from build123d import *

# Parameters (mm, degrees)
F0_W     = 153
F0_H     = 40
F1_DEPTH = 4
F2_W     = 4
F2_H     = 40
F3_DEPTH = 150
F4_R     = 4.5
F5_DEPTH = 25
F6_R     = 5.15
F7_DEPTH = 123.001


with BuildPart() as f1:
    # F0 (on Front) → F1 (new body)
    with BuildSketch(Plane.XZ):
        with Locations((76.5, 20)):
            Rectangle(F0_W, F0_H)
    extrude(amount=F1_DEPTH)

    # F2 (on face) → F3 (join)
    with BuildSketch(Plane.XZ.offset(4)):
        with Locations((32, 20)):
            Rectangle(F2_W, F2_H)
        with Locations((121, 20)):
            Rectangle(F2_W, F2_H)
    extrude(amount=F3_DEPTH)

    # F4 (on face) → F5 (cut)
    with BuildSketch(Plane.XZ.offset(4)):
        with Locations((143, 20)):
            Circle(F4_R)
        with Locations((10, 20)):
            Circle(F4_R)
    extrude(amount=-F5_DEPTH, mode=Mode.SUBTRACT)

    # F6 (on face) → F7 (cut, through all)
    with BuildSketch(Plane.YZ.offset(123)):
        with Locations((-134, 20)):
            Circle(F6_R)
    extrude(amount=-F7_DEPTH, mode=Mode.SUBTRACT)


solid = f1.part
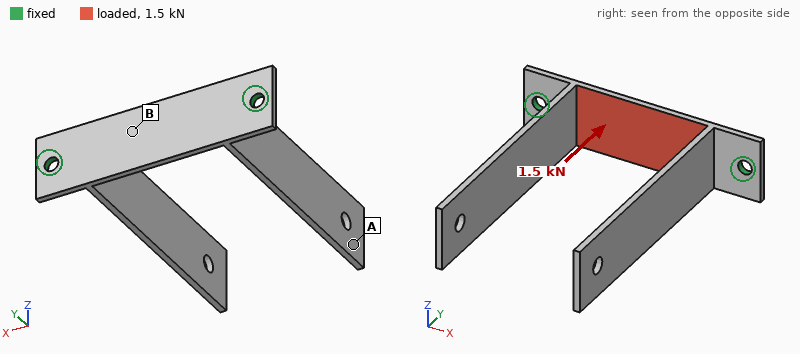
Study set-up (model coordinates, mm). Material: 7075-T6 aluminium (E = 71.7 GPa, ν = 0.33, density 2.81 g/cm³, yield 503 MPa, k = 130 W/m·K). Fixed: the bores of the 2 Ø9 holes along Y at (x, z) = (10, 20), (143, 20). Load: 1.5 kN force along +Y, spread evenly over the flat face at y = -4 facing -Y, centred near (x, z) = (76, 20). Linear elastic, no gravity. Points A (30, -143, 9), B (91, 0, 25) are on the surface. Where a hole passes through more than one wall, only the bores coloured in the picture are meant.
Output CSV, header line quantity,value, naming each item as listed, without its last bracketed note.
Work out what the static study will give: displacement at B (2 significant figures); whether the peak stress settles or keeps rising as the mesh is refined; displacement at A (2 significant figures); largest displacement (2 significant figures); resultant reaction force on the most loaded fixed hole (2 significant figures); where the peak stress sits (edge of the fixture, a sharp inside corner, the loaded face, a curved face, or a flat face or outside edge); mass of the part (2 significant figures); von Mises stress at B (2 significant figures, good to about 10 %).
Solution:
quantity,value
displacement at B,0.69 mm
whether the peak stress settles or keeps rising as the mesh is refined,keeps rising
displacement at A,2.4 mm
largest displacement,2.6 mm
resultant reaction force on the most loaded fixed hole,750 N
where the peak stress sits,edge of the fixture
mass of the part,200 g
von Mises stress at B,87 MPa
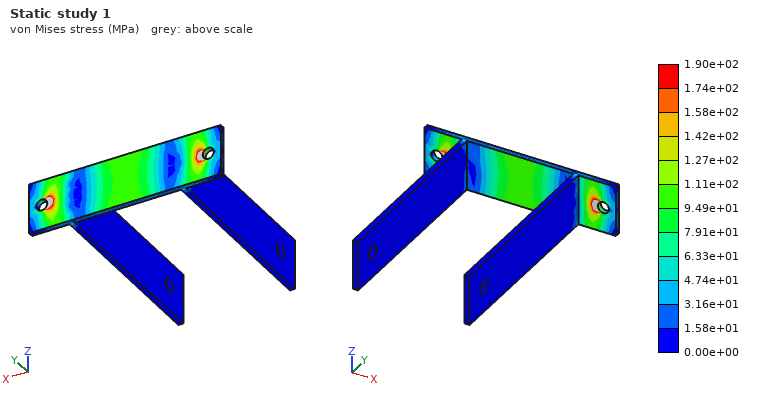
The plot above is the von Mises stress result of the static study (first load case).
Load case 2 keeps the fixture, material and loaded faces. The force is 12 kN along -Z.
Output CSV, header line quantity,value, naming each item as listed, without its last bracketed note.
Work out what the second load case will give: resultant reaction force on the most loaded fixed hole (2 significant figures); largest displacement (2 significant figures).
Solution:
quantity,value
resultant reaction force on the most loaded fixed hole,6.0 kN
largest displacement,1.4 mm
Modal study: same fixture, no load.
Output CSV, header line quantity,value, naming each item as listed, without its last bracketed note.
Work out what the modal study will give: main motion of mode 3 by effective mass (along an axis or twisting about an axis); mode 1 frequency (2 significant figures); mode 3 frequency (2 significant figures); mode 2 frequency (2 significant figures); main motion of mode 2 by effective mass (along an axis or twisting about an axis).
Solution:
quantity,value
main motion of mode 3 by effective mass,along Z
mode 1 frequency,130 Hz
mode 3 frequency,280 Hz
mode 2 frequency,140 Hz
main motion of mode 2 by effective mass,along X
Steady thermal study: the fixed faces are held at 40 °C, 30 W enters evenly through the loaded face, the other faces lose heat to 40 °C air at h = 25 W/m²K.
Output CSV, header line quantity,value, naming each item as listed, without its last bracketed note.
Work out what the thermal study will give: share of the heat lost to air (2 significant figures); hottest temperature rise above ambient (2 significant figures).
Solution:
quantity,value
share of the heat lost to air,27 %
hottest temperature rise above ambient,28 K
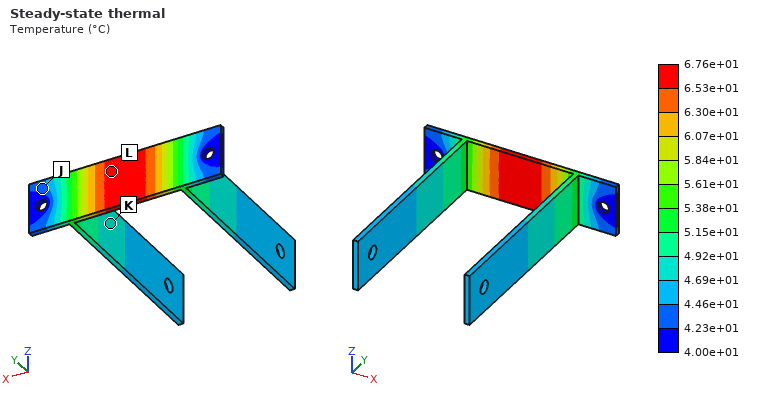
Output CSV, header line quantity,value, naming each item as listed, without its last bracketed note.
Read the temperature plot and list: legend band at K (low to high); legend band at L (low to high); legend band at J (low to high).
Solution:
quantity,value
legend band at K,4.69e+01 to 4.92e+01 °C
legend band at L,6.53e+01 to 6.76e+01 °C
legend band at J,4.23e+01 to 4.46e+01 °C
